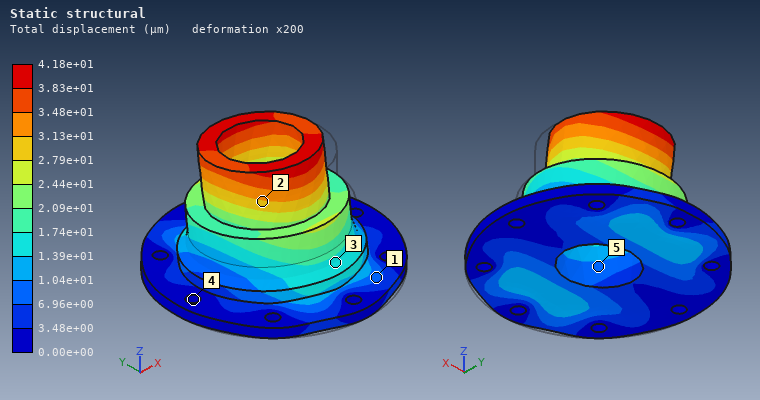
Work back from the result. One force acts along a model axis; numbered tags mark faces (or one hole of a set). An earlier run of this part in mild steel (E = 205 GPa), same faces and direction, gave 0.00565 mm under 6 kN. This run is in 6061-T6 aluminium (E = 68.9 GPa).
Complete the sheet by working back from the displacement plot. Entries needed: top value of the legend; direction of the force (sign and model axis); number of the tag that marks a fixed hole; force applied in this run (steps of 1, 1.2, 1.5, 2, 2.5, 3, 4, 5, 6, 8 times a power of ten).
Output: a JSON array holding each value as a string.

["4.18e+01 µm", "+Y", "4", "15 kN"]
